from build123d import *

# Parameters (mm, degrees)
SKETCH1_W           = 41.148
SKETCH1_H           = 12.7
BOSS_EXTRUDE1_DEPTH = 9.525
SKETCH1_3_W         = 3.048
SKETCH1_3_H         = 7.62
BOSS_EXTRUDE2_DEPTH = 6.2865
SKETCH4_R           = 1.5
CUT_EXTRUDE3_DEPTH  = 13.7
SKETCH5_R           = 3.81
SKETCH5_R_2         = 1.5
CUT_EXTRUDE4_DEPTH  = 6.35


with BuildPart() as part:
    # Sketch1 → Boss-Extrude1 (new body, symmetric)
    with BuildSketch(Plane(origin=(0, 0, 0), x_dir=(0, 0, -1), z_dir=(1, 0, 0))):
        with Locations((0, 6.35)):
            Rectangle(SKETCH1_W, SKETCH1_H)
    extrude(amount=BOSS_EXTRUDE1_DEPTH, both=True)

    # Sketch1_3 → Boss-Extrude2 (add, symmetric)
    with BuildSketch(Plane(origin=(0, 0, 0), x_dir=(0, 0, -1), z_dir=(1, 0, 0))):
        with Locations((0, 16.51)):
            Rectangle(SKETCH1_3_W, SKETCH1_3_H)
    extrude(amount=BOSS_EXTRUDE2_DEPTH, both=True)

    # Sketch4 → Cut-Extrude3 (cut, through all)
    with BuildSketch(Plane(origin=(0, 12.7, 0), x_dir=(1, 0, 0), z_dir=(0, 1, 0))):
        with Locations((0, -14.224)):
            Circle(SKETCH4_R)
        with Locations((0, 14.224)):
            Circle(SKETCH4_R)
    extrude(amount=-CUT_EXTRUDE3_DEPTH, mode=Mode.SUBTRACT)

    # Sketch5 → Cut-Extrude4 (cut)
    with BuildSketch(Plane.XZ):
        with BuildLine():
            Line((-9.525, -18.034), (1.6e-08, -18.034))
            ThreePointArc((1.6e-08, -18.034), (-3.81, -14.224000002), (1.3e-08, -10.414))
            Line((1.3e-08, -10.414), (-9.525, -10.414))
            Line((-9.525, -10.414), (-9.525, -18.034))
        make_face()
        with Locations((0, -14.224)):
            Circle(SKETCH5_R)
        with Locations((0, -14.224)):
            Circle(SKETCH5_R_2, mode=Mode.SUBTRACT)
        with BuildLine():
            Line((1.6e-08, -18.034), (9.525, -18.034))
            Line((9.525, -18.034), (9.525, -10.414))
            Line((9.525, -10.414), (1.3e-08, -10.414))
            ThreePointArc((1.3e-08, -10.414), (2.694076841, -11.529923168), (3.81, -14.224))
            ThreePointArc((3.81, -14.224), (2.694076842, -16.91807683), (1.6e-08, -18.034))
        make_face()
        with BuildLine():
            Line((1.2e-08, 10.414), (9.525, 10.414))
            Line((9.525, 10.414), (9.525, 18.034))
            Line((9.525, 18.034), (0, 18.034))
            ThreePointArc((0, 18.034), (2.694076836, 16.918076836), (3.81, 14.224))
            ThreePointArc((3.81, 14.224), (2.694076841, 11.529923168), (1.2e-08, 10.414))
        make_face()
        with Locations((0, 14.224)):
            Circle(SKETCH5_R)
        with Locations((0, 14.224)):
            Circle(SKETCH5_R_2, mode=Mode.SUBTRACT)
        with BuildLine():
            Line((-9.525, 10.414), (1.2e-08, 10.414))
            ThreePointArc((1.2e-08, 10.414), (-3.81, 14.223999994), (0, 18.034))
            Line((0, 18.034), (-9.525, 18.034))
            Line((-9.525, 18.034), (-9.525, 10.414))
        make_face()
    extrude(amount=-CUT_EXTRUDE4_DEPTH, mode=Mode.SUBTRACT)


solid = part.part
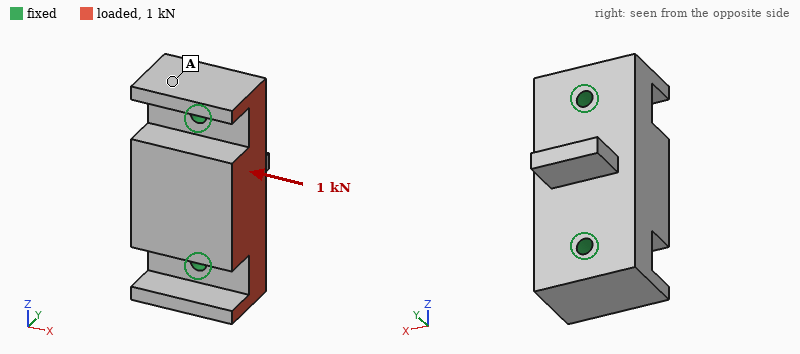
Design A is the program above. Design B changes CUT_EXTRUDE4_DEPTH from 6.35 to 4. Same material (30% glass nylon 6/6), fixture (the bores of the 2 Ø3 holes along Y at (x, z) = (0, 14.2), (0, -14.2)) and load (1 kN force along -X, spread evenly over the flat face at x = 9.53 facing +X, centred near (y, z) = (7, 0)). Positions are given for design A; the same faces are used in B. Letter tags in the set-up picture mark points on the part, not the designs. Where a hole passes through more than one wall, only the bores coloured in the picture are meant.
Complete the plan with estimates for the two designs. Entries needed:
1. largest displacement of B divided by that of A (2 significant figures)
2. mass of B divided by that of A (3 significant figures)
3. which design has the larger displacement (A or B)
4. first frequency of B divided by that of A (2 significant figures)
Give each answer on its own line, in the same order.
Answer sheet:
0.43
1.08
A
1.4
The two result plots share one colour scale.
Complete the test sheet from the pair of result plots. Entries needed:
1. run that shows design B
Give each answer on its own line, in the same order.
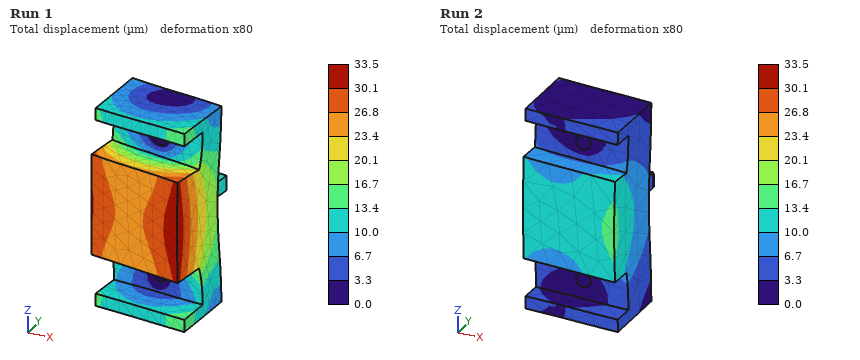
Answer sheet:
Run 2
